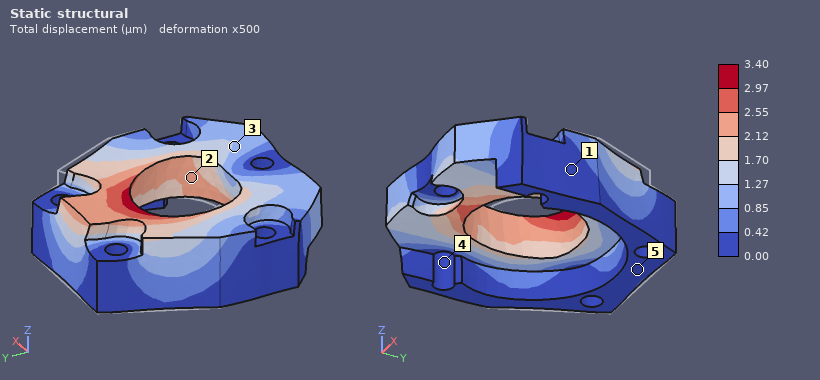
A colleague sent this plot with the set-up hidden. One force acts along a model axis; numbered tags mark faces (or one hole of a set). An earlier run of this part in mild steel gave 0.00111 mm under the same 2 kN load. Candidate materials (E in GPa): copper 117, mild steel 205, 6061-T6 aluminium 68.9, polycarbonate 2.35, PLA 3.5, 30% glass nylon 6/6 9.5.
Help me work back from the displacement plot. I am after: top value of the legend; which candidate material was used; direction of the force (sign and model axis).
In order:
3.40 µm
6061-T6 aluminium
-Y
